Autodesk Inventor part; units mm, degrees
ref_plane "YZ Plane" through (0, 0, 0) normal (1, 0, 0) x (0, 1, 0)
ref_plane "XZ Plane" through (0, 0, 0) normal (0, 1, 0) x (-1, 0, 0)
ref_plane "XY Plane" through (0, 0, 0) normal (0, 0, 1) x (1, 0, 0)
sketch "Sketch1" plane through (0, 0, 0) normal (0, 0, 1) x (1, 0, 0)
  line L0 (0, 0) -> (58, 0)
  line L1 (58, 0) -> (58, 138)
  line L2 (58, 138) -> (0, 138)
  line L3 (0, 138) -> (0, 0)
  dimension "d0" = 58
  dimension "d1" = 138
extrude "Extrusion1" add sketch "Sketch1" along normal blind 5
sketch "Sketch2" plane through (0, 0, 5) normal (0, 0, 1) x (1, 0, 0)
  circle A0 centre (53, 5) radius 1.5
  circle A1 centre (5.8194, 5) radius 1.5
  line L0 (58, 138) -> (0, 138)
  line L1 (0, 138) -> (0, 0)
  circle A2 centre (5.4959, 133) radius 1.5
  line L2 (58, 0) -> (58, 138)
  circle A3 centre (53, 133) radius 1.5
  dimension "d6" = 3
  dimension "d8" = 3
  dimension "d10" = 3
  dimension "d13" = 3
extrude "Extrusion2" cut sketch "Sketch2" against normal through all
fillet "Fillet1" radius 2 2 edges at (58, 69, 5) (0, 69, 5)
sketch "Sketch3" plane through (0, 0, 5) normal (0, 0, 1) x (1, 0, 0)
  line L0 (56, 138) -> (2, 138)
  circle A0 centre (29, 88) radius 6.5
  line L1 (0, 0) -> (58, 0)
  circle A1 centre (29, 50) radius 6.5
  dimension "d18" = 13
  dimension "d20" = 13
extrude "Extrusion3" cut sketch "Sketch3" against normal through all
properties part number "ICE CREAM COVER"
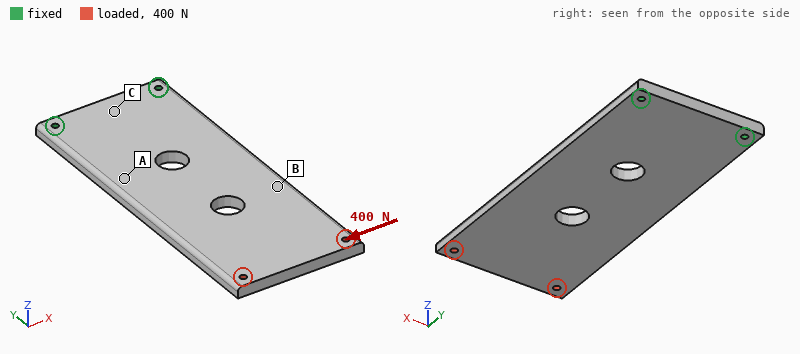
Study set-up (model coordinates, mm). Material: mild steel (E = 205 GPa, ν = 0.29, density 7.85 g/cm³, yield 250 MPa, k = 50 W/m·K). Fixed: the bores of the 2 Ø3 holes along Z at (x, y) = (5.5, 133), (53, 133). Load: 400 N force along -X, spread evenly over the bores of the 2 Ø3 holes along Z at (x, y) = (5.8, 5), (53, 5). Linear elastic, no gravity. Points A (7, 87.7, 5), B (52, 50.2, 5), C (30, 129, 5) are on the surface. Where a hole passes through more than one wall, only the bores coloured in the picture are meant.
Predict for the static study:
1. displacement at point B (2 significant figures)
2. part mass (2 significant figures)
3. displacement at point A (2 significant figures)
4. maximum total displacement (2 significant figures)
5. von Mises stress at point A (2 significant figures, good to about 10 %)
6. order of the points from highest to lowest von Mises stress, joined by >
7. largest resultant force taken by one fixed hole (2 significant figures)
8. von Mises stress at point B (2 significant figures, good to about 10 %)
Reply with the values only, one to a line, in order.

12 µm
300 g
5.3 µm
24 µm
9.4 MPa
A > B > C
1.1 kN
5.6 MPa
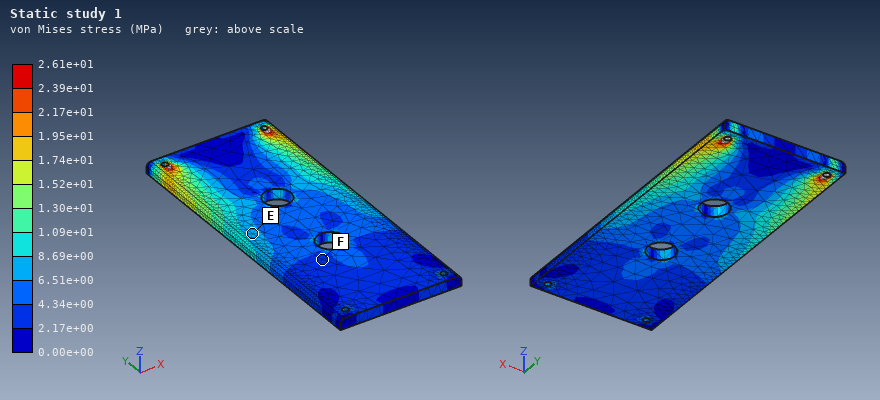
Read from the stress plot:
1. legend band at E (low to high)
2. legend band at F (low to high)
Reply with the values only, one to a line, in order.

6.51e+00 to 8.69e+00 MPa
2.17e+00 to 4.34e+00 MPa
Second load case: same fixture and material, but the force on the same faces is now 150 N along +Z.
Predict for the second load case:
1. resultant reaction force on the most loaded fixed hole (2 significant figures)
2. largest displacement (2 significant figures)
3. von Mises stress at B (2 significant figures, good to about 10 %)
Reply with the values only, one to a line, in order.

78 N
1.1 mm
34 MPa
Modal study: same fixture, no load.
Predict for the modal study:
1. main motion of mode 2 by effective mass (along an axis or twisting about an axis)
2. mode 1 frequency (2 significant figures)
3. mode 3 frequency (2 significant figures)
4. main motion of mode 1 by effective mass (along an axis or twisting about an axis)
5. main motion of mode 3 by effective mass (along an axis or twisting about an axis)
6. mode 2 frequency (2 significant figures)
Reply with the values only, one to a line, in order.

twisting about Y
210 Hz
1300 Hz
along Z
along Z
1100 Hz
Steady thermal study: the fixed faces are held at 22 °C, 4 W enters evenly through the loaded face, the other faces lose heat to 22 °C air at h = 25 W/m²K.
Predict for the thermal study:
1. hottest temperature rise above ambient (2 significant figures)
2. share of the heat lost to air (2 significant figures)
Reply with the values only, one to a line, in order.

21 K
78 %
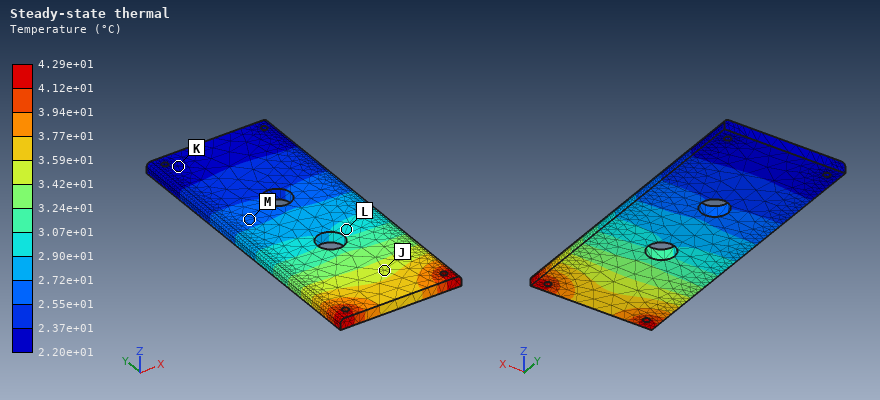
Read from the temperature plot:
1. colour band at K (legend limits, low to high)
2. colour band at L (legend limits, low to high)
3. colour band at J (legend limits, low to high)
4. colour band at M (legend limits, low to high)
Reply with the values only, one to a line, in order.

2.20e+01 to 2.37e+01 °C
2.90e+01 to 3.07e+01 °C
3.42e+01 to 3.59e+01 °C
2.55e+01 to 2.72e+01 °C
